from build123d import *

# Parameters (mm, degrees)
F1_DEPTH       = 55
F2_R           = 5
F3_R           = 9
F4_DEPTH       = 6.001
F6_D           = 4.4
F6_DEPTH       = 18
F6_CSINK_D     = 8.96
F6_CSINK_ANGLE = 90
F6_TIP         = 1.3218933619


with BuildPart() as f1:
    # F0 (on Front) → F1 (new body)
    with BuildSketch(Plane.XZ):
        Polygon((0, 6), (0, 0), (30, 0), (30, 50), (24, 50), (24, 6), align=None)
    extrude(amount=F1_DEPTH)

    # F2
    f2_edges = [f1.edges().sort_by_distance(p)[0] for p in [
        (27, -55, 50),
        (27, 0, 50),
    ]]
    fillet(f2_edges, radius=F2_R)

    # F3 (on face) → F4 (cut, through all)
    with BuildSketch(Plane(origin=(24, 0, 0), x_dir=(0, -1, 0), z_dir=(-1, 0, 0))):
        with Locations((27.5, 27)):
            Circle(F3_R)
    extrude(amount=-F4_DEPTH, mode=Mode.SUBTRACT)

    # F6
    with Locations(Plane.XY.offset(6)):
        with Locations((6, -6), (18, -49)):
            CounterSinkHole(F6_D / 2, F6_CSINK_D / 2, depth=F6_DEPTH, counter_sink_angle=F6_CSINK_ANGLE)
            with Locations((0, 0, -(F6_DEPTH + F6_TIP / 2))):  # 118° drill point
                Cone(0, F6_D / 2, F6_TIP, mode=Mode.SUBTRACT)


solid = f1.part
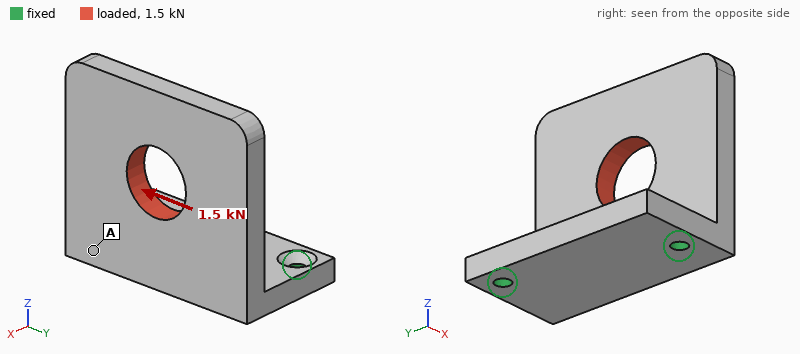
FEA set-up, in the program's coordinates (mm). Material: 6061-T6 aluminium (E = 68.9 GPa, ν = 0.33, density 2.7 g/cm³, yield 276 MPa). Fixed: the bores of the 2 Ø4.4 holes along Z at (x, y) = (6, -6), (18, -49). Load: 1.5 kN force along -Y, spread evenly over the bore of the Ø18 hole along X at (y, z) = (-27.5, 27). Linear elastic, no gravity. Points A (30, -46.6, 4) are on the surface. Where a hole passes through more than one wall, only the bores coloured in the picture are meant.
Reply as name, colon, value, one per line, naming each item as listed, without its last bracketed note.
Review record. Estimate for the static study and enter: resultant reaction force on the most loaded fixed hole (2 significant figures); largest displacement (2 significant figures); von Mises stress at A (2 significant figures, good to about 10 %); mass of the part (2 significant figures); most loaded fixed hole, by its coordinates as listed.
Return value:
resultant reaction force on the most loaded fixed hole: 1.3 kN
largest displacement: 0.21 mm
von Mises stress at A: 26 MPa
mass of the part: 61 g
most loaded fixed hole, by its coordinates as listed: (18, -49)
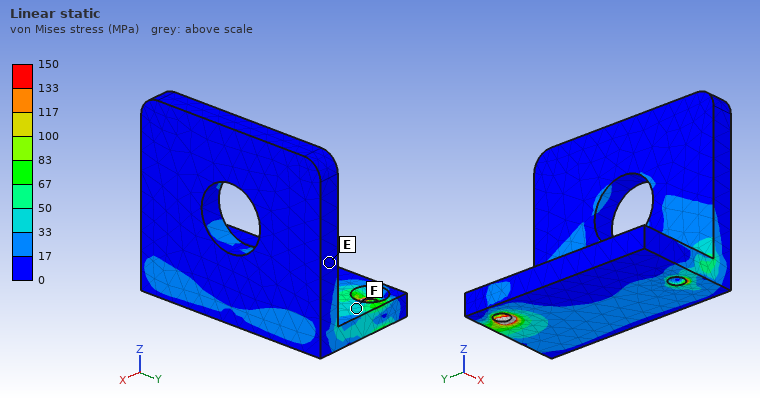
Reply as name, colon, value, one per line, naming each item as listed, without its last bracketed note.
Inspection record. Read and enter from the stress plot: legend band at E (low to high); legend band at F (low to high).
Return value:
legend band at E: 0 to 17 MPa
legend band at F: 33 to 50 MPa
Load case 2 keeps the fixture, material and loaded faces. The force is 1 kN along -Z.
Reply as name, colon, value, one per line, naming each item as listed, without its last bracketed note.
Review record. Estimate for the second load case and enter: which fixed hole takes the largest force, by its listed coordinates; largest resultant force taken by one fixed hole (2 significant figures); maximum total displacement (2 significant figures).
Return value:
which fixed hole takes the largest force, by its listed coordinates: (18, -49)
largest resultant force taken by one fixed hole: 590 N
maximum total displacement: 0.18 mm
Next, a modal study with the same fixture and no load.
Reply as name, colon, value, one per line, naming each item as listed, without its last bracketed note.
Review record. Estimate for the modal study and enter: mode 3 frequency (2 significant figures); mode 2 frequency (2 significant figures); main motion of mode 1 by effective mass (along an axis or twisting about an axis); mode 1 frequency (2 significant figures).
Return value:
mode 3 frequency: 4200 Hz
mode 2 frequency: 3000 Hz
main motion of mode 1 by effective mass: along X
mode 1 frequency: 1300 Hz
